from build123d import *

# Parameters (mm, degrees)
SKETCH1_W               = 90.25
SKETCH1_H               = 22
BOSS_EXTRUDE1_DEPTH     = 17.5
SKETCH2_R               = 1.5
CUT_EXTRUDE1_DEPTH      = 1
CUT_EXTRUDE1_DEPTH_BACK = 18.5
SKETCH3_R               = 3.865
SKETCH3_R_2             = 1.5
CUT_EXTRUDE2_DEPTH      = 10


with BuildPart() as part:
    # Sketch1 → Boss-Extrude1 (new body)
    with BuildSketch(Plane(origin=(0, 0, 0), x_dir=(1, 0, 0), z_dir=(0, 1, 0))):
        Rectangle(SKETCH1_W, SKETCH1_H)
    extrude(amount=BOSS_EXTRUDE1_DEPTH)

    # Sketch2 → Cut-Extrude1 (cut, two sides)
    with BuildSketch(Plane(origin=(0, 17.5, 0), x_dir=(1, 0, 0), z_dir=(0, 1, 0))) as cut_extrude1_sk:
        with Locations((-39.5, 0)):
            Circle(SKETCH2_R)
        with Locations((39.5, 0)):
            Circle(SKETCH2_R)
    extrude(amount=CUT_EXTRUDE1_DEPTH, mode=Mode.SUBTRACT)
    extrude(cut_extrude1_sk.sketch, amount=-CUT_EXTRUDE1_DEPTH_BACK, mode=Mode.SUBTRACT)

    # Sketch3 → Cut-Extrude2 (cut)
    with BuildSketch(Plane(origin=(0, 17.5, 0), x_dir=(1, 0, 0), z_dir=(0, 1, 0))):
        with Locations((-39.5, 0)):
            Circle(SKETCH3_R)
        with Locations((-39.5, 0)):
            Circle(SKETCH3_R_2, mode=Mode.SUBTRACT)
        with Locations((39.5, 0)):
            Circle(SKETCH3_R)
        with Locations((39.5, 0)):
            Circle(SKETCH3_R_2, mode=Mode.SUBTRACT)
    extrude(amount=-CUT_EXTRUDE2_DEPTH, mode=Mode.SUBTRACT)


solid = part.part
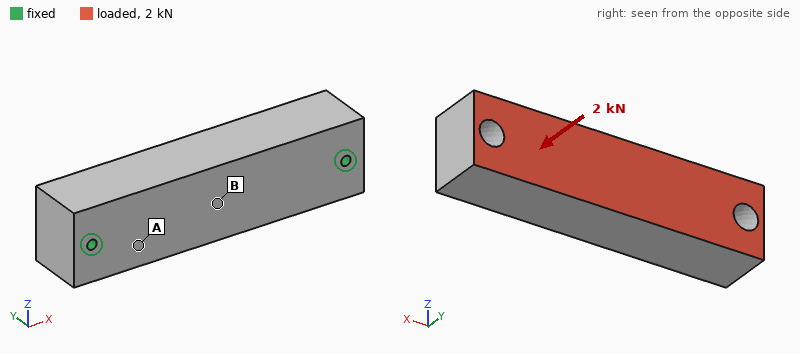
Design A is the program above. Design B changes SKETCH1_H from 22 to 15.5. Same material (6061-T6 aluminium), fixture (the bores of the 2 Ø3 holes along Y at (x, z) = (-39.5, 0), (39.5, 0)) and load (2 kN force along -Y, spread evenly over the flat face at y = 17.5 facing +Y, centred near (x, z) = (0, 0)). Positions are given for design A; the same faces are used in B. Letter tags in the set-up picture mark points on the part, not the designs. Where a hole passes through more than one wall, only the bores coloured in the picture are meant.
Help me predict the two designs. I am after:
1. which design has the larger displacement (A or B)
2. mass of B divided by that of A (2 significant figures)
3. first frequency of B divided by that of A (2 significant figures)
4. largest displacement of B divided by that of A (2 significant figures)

B
0.70
0.94
1.3
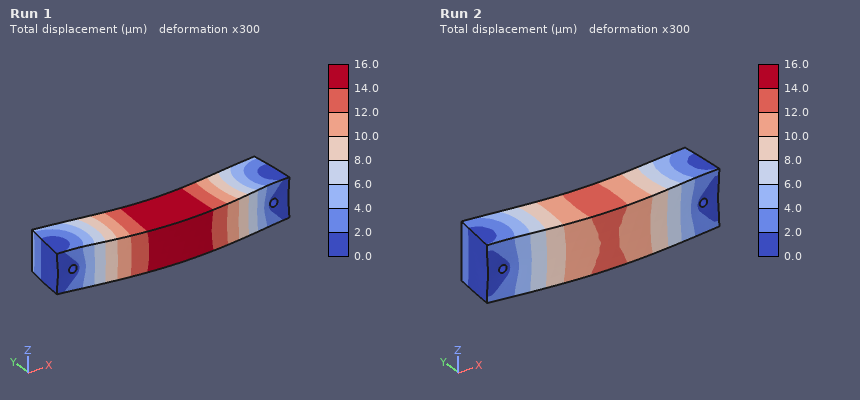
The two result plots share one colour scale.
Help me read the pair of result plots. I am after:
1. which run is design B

Run 1
